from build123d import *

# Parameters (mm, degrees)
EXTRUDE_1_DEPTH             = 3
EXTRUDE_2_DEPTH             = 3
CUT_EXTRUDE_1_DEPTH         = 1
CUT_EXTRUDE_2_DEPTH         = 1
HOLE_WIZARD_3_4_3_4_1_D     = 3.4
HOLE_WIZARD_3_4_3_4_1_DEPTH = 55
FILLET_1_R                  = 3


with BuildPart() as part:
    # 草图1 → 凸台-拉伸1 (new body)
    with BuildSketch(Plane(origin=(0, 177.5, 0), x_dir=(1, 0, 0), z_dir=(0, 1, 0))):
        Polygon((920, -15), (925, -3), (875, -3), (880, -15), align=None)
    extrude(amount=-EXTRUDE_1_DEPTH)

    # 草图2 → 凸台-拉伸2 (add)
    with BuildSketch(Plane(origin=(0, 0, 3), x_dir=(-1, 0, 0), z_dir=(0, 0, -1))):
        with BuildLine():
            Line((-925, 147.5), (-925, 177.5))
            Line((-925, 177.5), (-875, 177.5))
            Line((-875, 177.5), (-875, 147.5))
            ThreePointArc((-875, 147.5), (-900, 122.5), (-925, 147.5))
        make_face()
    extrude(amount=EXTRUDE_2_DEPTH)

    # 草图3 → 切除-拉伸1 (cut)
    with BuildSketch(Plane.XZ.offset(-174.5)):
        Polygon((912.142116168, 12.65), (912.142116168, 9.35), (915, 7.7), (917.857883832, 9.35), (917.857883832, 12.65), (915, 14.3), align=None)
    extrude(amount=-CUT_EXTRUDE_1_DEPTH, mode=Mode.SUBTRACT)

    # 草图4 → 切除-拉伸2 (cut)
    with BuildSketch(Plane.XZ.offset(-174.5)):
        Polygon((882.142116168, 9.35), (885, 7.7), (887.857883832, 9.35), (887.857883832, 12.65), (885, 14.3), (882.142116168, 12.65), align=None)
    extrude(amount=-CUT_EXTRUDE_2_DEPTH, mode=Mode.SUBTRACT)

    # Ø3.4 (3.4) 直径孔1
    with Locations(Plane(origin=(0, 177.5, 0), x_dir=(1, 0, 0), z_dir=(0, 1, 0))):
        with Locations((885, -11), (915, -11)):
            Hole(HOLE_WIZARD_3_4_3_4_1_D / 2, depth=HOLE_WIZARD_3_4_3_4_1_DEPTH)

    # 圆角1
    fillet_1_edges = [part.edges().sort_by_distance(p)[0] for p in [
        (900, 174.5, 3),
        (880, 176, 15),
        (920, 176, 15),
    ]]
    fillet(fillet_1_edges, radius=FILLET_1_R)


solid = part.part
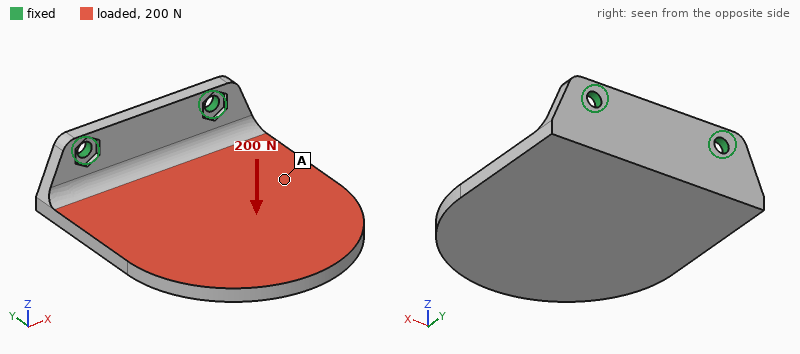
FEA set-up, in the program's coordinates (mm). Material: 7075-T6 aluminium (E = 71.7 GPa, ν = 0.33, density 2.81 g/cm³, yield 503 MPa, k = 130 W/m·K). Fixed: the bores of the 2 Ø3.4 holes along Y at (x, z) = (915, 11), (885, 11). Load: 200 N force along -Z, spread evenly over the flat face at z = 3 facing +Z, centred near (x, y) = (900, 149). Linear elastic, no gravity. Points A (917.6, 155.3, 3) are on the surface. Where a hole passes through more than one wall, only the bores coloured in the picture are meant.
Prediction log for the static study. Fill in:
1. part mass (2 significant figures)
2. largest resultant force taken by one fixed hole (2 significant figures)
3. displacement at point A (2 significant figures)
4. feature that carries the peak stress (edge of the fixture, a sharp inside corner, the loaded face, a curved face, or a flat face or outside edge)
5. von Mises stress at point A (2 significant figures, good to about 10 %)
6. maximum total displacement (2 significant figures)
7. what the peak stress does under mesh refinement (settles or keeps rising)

25 g
140 N
0.27 mm
edge of the fixture
23 MPa
0.86 mm
keeps rising
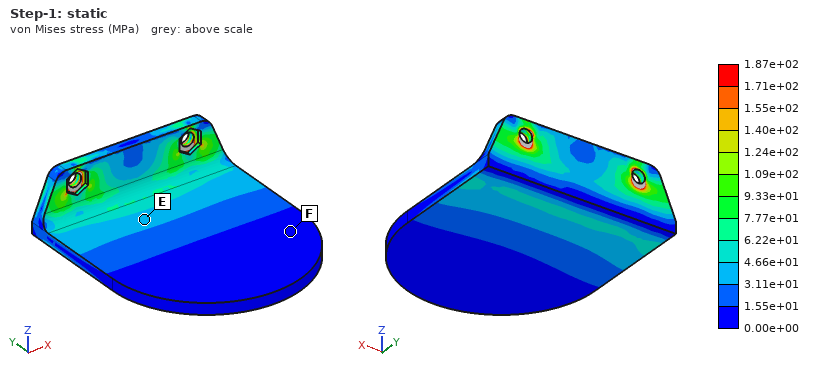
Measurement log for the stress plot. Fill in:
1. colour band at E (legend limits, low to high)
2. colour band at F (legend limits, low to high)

3.11e+01 to 4.66e+01 MPa
0.00e+00 to 1.55e+01 MPa
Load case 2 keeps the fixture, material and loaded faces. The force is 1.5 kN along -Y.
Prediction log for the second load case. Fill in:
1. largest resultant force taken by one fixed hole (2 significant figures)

750 N
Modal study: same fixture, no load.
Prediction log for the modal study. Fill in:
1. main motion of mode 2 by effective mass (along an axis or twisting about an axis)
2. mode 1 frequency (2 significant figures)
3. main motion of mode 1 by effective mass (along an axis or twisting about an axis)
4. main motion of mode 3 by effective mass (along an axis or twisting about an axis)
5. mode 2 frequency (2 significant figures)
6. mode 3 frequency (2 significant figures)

along X
730 Hz
along Z
along X
2200 Hz
3400 Hz
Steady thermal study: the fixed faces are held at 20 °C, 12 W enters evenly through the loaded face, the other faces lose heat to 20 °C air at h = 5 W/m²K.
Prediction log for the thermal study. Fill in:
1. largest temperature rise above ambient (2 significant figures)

24 K
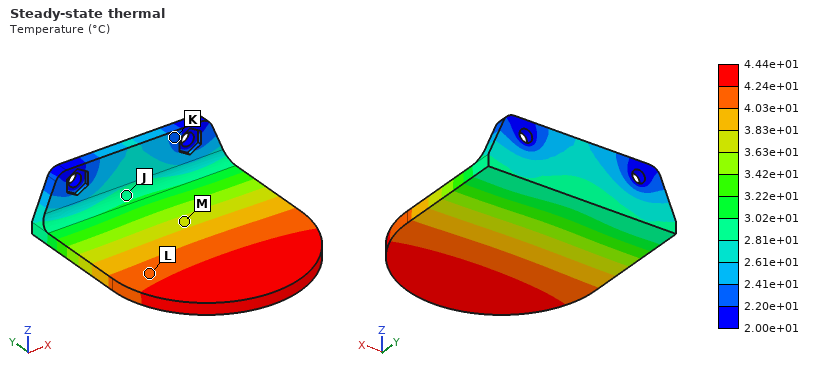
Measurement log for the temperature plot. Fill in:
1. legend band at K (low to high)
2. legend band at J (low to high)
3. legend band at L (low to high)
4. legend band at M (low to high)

2.20e+01 to 2.41e+01 °C
2.81e+01 to 3.02e+01 °C
4.03e+01 to 4.24e+01 °C
3.63e+01 to 3.83e+01 °C
